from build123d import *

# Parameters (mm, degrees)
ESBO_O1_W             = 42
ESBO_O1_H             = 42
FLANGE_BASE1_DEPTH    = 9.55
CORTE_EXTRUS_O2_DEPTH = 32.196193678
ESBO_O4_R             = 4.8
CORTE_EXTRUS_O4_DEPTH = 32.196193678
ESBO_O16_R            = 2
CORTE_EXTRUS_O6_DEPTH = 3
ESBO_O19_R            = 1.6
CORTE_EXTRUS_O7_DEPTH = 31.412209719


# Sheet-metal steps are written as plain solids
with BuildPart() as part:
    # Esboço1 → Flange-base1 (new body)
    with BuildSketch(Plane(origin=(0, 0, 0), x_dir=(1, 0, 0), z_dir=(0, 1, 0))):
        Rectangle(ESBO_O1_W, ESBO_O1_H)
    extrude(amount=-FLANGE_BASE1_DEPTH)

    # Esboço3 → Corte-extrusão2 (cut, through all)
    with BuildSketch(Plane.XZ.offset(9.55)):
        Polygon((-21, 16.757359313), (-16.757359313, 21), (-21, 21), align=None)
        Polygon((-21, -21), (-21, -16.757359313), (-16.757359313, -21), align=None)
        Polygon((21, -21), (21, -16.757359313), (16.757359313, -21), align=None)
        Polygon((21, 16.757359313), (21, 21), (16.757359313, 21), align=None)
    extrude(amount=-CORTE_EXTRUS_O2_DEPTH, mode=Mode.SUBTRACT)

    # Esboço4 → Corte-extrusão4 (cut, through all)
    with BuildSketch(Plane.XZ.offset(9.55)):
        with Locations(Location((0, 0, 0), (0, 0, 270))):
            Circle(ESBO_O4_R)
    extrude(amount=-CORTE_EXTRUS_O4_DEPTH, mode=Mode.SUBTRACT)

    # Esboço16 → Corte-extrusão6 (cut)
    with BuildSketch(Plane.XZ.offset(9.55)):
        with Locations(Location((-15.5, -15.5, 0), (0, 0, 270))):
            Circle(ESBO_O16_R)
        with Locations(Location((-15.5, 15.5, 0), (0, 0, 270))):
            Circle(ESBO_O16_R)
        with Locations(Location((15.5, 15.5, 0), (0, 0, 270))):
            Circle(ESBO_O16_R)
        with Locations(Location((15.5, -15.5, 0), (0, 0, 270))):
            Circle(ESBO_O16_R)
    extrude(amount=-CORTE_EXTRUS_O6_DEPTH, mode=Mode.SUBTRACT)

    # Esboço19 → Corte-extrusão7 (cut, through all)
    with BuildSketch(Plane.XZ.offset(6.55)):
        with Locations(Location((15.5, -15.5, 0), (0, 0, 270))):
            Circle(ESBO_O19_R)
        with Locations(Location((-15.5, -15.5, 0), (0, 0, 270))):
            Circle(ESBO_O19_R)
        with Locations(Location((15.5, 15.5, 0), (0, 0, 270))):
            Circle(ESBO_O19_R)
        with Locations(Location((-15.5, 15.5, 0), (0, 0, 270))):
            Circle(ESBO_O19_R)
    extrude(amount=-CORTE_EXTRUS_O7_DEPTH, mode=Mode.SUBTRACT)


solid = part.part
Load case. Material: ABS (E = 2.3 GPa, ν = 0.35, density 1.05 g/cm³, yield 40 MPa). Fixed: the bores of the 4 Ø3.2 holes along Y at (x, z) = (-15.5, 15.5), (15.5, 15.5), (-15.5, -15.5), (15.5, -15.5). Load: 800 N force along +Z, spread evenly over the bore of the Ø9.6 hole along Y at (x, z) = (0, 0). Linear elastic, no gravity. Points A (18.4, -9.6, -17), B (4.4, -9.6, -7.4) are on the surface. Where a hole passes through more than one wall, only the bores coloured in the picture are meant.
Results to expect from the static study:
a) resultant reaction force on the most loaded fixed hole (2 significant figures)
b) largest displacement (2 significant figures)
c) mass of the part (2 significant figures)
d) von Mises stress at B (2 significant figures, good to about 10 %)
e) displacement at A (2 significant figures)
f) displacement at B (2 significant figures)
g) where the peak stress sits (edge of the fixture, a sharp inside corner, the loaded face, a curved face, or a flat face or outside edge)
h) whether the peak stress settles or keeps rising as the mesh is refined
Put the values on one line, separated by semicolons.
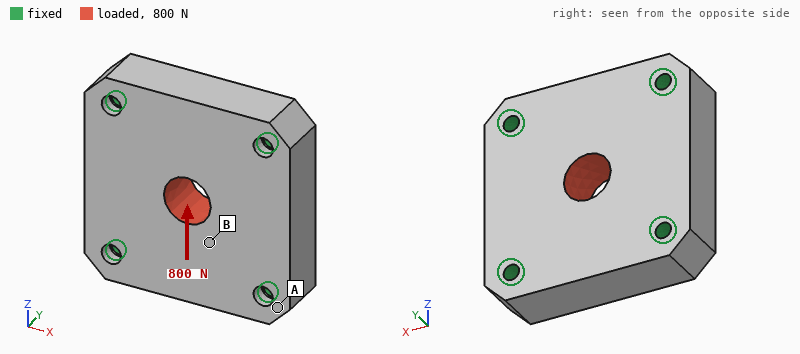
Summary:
220 N; 27 µm; 16 g; 2.3 MPa; 4.4 µm; 20 µm; edge of the fixture; keeps rising
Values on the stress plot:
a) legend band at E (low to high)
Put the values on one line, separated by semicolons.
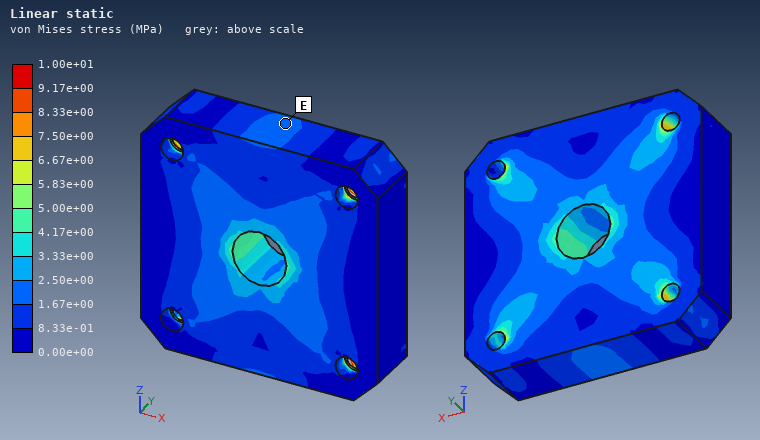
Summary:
1.67e+00 to 2.50e+00 MPa
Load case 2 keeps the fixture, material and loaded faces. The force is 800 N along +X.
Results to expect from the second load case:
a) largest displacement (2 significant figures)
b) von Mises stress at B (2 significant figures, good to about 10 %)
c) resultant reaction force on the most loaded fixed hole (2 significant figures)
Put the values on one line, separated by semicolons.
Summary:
27 µm; 2.1 MPa; 220 N
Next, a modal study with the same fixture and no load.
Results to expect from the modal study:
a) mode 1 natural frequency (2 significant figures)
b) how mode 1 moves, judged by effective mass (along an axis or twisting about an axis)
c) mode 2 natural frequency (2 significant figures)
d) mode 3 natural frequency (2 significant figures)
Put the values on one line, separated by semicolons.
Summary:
6600 Hz; along Y; 9300 Hz; 9300 Hz
